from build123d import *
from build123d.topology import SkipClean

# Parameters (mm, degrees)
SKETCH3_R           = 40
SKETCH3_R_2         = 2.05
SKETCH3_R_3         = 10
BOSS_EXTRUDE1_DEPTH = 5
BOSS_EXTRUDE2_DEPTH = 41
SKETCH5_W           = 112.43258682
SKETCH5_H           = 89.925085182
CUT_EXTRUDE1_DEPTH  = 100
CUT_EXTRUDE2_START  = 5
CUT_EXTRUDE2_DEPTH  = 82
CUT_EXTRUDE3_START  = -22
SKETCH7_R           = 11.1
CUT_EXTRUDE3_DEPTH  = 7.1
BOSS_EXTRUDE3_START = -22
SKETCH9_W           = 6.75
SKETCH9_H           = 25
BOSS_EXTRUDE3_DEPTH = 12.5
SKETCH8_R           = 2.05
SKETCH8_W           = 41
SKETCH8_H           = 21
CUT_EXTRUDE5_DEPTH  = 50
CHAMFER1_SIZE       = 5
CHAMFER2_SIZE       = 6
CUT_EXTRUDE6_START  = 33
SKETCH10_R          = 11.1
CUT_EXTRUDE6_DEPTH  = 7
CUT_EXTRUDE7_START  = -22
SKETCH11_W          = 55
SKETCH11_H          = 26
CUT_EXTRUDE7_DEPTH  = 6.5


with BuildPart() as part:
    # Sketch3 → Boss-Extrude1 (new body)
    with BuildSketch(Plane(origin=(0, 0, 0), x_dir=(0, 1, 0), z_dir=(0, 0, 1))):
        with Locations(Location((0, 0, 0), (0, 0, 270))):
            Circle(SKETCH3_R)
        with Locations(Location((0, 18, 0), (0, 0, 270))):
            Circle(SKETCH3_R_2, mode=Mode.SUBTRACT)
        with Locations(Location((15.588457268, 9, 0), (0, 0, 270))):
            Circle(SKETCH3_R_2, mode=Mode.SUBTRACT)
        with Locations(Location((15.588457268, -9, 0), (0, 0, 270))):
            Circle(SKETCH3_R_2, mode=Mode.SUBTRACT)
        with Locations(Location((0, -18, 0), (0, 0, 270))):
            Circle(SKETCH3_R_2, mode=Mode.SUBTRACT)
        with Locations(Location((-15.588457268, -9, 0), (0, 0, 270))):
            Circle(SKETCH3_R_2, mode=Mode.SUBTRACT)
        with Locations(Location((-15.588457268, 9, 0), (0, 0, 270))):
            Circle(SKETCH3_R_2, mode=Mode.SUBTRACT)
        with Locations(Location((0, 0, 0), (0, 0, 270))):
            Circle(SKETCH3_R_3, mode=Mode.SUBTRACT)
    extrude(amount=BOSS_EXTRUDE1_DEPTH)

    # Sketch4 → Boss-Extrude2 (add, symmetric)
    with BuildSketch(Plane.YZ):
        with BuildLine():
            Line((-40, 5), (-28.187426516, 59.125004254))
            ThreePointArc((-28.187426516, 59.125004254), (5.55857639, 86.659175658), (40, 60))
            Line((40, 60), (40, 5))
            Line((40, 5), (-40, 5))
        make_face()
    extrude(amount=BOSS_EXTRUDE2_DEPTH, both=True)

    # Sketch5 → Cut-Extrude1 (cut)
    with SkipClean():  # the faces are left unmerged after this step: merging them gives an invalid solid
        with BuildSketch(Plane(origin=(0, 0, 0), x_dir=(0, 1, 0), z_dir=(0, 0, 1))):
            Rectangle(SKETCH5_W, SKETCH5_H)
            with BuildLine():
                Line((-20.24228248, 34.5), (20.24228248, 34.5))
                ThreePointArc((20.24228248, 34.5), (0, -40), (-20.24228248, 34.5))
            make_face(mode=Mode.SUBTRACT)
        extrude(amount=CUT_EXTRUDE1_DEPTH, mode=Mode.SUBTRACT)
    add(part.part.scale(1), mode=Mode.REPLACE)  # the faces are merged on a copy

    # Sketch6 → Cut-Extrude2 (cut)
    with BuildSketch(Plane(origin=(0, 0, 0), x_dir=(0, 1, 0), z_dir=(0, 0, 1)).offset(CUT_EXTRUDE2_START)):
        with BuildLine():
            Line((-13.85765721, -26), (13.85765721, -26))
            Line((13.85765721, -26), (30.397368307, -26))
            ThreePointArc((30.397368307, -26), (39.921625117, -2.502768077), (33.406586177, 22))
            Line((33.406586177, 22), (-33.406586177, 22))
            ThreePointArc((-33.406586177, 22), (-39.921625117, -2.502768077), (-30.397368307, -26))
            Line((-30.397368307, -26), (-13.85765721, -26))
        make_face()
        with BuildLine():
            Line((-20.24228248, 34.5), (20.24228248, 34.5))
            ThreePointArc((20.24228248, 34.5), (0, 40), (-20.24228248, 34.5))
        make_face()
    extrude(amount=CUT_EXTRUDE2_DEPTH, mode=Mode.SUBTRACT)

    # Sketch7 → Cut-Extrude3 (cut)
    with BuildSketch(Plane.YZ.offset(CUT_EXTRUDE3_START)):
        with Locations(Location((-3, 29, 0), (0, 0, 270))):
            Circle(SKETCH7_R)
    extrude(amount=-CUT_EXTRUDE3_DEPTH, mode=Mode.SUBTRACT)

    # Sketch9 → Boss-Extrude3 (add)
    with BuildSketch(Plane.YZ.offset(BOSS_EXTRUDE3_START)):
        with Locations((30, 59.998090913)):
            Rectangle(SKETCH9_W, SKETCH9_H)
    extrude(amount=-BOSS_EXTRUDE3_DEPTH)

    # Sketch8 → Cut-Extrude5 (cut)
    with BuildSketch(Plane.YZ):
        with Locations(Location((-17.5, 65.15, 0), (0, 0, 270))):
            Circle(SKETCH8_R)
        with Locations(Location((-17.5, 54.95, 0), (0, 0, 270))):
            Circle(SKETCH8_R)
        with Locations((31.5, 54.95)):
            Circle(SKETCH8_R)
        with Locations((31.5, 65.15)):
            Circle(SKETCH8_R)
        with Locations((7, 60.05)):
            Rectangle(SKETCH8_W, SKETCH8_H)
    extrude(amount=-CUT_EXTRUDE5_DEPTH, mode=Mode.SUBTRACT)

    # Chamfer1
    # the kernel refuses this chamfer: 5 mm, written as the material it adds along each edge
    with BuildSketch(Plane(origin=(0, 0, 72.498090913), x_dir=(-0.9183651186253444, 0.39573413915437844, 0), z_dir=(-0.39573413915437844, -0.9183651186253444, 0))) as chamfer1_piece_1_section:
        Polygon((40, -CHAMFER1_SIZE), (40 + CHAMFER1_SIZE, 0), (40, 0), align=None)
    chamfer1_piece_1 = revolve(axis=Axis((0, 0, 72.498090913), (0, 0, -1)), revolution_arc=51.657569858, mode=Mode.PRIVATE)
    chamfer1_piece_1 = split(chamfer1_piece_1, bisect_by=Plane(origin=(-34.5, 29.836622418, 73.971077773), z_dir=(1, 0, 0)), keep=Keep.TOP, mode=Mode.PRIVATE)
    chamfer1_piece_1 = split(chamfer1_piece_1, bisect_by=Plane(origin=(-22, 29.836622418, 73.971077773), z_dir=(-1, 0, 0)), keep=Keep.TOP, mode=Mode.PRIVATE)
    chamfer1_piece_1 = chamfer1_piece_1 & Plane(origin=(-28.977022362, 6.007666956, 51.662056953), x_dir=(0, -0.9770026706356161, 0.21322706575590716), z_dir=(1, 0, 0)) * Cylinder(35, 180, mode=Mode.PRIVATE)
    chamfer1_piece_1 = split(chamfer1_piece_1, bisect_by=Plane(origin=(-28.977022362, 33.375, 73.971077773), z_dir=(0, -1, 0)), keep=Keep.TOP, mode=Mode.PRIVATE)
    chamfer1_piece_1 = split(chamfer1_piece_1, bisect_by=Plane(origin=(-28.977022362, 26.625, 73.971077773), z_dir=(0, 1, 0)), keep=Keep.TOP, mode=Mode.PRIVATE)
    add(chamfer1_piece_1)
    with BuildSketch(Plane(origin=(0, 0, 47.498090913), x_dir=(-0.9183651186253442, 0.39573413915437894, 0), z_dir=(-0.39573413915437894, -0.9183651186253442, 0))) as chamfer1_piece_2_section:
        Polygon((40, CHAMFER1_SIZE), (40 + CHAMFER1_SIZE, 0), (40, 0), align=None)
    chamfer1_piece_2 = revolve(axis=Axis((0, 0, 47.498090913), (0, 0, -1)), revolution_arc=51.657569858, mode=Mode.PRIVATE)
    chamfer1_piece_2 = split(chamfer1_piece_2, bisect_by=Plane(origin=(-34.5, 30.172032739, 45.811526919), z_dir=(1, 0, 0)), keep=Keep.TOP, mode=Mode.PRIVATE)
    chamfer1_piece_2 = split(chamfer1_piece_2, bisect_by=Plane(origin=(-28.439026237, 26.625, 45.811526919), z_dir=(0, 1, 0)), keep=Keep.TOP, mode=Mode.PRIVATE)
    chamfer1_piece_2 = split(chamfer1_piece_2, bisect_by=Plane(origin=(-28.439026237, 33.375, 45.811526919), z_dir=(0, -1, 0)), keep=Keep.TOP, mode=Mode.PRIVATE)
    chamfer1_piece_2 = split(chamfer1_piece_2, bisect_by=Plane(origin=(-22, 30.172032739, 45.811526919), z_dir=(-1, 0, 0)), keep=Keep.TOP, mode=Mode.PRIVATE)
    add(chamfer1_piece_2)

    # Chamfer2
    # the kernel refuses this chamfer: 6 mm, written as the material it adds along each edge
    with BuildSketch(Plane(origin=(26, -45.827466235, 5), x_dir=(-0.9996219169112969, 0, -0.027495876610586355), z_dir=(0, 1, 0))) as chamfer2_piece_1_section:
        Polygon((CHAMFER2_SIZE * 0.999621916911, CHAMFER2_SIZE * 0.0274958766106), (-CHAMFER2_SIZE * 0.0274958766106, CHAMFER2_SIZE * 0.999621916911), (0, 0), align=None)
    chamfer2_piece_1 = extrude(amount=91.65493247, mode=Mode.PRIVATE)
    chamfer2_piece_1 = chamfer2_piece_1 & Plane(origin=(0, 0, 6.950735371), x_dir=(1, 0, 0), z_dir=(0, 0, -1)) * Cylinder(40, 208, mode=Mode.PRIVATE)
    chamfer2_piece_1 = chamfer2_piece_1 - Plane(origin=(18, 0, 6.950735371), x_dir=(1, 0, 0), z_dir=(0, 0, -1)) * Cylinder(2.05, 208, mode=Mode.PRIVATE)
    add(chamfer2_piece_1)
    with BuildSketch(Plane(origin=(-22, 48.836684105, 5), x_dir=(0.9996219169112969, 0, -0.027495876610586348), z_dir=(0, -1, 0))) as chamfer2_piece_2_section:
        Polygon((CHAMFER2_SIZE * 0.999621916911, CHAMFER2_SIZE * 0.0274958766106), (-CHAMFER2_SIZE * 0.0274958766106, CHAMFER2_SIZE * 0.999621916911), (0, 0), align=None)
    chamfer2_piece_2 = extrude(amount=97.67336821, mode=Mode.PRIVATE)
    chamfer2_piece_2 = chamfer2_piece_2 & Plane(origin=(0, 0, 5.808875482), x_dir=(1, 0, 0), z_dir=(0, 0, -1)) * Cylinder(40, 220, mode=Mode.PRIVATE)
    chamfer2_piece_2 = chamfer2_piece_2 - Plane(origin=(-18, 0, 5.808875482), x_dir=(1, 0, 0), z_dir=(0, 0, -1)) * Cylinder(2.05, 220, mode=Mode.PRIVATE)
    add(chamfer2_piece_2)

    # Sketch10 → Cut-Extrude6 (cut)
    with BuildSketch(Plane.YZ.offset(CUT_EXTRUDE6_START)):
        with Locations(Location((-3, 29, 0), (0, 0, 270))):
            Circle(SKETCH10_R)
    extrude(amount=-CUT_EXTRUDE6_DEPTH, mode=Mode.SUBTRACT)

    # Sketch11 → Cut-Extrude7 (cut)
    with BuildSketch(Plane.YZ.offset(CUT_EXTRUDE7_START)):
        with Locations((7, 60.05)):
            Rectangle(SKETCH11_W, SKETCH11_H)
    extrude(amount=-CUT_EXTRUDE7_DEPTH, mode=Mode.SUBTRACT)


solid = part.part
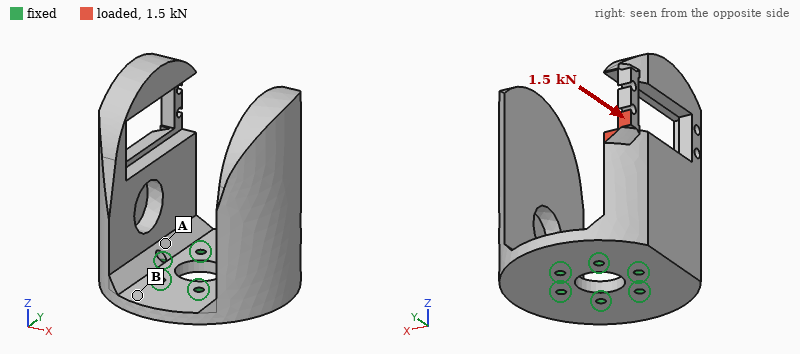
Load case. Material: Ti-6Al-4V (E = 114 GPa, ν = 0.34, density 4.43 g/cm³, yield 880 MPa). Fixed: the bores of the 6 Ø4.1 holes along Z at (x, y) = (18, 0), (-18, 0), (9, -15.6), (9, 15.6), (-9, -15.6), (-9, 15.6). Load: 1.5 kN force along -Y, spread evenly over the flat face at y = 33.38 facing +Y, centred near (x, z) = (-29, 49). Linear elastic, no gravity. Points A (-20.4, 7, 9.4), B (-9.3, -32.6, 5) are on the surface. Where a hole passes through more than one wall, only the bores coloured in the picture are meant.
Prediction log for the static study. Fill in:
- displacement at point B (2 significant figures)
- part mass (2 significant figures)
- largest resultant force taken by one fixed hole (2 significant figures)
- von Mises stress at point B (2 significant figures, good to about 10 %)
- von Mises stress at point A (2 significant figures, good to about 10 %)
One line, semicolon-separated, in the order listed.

0.019 mm; 470 g; 1.8 kN; 17 MPa; 44 MPa
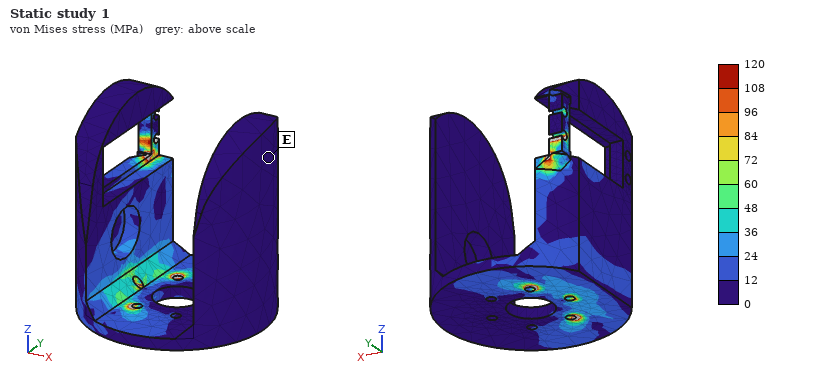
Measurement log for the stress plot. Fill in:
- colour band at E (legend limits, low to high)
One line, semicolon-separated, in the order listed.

0 to 12 MPa
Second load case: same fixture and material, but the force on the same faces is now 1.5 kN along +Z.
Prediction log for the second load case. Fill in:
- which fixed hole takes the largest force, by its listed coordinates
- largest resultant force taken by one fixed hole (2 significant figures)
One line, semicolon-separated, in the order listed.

(-18, 0); 1.9 kN
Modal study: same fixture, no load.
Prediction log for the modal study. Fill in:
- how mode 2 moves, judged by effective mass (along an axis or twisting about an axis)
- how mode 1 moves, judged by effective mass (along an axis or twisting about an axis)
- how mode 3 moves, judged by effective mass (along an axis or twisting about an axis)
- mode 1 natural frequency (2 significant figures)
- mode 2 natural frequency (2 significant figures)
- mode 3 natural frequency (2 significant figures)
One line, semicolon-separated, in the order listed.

along X; along X; along Y; 660 Hz; 910 Hz; 1400 Hz
